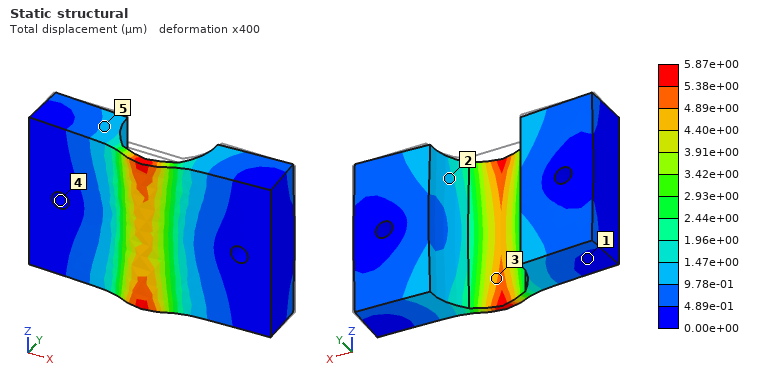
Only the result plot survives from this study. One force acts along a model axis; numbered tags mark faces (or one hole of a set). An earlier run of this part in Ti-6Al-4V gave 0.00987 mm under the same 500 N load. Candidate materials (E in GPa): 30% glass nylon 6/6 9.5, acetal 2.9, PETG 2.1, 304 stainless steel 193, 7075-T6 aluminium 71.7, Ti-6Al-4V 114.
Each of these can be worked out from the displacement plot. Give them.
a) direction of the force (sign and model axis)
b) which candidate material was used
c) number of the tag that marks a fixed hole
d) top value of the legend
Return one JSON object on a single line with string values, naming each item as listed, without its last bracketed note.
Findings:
{"direction of the force": "-Y", "which candidate material was used": "304 stainless steel", "number of the tag that marks a fixed hole": "4", "top value of the legend": "5.87e+00 µm"}
